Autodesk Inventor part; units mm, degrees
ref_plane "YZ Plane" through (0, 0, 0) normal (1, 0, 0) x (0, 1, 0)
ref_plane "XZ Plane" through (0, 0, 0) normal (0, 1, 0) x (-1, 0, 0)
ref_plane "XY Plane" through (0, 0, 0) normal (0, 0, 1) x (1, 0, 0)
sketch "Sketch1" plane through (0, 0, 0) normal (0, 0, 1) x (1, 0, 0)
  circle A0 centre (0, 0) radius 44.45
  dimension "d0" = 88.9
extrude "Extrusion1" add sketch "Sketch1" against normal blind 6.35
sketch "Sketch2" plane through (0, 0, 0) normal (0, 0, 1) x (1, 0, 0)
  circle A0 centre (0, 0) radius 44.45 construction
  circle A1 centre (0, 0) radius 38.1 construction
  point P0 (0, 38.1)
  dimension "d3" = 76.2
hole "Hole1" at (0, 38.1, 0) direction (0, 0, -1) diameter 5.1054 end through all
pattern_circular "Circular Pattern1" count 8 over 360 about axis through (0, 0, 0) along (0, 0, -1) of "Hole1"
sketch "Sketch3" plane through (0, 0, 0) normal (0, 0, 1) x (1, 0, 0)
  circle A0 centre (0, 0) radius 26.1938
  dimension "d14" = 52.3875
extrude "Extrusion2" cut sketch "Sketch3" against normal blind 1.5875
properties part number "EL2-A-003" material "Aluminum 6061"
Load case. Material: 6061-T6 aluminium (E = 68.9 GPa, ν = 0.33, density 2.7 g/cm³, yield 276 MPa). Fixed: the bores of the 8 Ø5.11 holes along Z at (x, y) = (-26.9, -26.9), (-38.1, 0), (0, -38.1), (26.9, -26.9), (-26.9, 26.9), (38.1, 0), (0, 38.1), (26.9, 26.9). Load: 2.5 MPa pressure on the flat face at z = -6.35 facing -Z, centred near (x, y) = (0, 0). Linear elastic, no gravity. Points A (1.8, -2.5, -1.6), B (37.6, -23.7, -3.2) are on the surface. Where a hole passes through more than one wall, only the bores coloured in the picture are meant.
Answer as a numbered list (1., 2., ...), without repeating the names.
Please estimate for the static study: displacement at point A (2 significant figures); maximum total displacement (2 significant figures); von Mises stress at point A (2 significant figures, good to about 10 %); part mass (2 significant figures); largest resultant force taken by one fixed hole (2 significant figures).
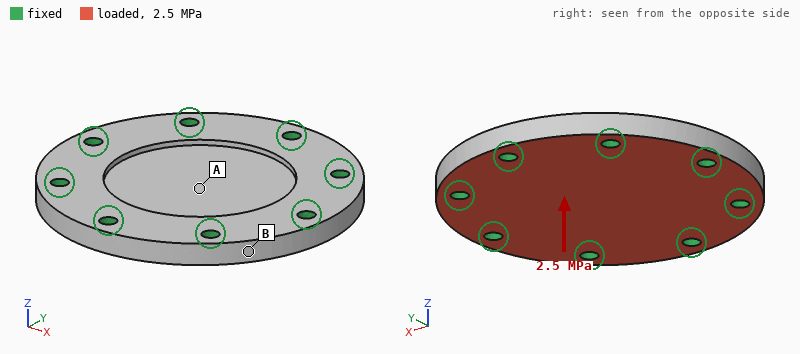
1. 89 µm
2. 90 µm
3. 58 MPa
4. 94 g
5. 2.0 kN
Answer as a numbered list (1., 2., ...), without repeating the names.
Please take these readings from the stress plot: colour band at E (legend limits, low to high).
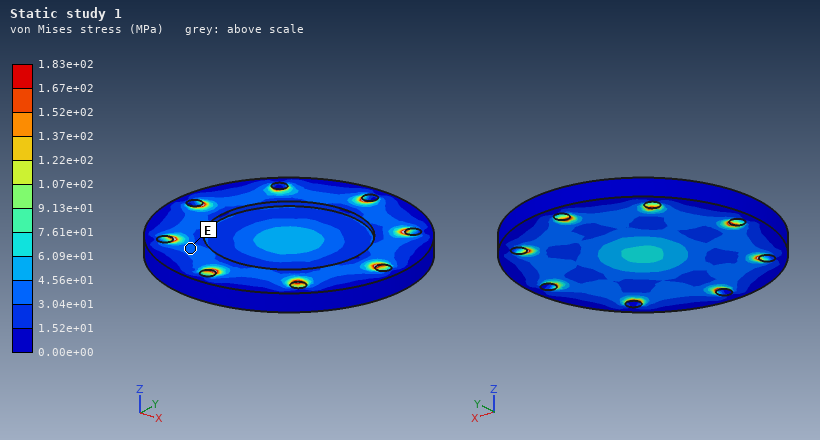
1. 3.04e+01 to 4.56e+01 MPa
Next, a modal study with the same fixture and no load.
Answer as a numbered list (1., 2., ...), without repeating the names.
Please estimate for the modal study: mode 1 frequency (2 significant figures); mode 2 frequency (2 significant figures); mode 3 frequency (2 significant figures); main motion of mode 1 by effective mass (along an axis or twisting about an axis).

1. 9200 Hz
2. 17 kHz
3. 17 kHz
4. along Z
